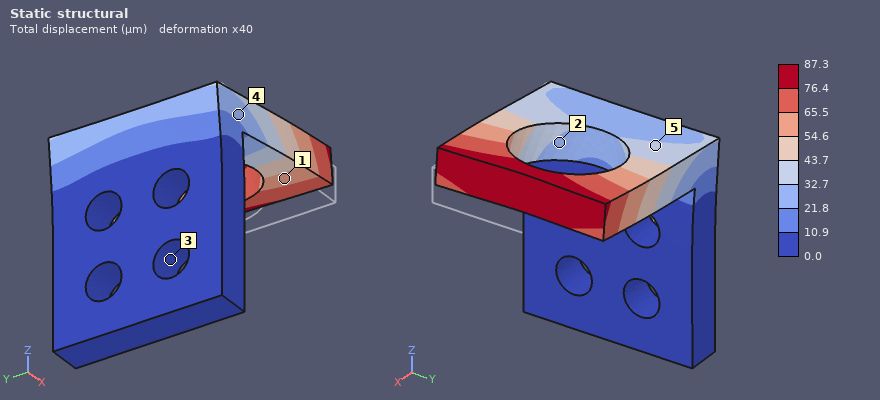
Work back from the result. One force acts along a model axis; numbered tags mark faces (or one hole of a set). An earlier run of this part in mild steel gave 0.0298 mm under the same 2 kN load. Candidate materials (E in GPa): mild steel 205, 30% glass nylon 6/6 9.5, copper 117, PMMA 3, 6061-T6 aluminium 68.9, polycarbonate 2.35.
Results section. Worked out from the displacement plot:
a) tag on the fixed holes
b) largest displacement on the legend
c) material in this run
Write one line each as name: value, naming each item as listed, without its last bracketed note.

tag on the fixed holes: 3
largest displacement on the legend: 87.3 µm
material in this run: 6061-T6 aluminium
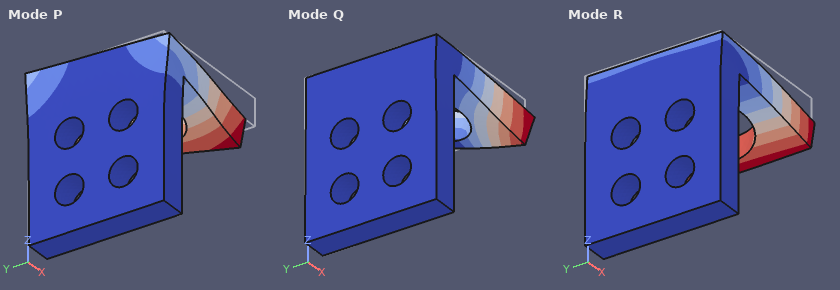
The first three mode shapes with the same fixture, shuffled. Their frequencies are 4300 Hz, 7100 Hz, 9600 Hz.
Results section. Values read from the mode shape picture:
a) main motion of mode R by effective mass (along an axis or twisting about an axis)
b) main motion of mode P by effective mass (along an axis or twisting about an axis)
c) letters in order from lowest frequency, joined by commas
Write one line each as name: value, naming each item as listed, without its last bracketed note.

main motion of mode R by effective mass: along Z
main motion of mode P by effective mass: along Y
letters in order from lowest frequency, joined by commas: R, P, Q
